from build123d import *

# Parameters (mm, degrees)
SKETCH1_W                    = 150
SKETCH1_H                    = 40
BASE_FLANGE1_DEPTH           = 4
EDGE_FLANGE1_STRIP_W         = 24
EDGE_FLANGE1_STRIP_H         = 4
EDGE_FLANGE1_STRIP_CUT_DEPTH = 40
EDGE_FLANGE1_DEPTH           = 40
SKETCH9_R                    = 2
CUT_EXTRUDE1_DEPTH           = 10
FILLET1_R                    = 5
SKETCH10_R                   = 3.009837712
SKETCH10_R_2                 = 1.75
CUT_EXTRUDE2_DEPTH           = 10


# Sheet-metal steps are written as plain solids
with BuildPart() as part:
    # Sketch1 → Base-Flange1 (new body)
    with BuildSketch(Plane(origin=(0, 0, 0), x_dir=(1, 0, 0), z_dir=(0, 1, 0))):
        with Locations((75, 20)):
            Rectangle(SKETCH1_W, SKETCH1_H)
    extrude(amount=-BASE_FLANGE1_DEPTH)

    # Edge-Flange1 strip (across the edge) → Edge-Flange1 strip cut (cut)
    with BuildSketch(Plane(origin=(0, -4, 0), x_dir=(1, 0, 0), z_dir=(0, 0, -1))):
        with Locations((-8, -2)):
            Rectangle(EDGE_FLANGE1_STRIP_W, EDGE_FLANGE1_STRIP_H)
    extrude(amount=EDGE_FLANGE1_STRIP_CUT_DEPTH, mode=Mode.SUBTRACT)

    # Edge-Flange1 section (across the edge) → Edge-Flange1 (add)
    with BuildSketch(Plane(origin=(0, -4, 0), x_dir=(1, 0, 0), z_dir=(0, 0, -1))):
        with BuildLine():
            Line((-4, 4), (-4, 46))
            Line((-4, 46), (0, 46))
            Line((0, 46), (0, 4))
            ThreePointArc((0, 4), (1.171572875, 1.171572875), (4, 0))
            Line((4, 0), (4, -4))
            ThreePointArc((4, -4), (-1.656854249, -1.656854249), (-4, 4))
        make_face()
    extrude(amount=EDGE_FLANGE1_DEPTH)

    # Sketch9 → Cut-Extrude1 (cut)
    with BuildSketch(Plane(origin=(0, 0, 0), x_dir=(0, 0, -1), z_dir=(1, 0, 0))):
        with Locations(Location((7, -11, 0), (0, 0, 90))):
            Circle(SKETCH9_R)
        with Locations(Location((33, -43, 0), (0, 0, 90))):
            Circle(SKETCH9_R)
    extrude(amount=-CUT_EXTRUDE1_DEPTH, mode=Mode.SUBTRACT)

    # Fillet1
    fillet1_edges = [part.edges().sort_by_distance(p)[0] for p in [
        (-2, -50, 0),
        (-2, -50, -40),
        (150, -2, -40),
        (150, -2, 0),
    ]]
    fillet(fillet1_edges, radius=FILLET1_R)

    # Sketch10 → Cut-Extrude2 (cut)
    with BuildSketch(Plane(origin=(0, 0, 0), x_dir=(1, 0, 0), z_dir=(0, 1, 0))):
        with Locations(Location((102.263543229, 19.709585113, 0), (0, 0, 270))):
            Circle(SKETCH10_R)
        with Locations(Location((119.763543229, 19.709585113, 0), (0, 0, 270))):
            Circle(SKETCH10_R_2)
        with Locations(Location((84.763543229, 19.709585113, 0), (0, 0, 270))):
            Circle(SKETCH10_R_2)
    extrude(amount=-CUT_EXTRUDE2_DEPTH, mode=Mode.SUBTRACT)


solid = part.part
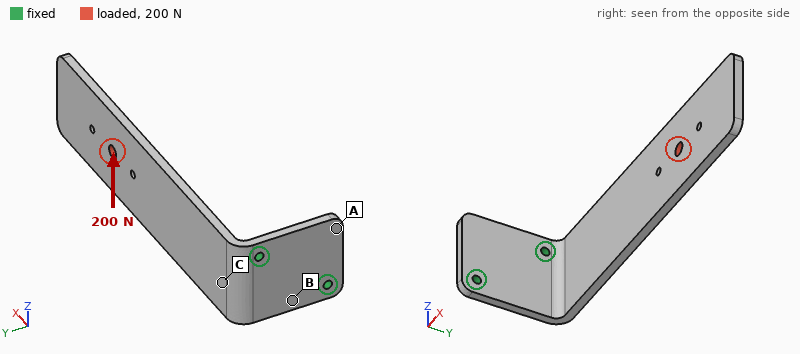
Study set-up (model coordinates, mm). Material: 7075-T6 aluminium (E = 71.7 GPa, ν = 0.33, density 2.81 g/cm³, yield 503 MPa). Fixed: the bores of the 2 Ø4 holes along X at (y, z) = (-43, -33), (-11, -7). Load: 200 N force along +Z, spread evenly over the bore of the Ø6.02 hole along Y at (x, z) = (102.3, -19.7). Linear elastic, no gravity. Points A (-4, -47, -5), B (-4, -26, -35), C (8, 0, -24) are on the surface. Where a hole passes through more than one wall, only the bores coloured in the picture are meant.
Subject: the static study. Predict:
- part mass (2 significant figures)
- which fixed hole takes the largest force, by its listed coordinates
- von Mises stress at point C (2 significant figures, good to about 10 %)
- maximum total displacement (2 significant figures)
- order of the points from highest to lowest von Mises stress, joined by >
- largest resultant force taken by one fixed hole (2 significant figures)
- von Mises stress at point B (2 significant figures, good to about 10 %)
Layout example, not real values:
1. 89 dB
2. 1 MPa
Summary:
1. 88 g
2. (-11, -7)
3. 36 MPa
4. 1.8 mm
5. B > C > A
6. 250 N
7. 59 MPa
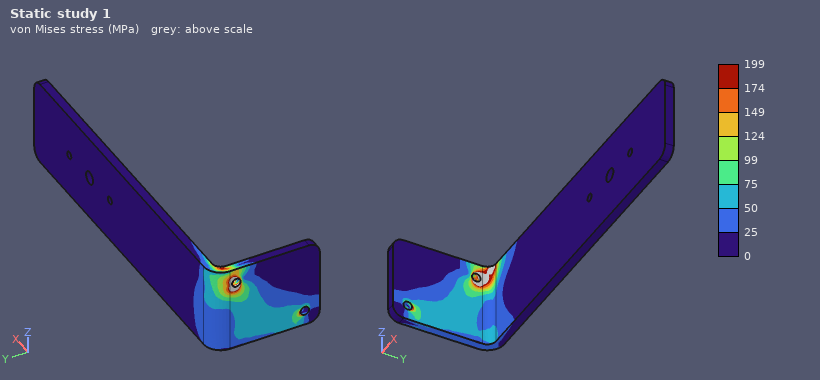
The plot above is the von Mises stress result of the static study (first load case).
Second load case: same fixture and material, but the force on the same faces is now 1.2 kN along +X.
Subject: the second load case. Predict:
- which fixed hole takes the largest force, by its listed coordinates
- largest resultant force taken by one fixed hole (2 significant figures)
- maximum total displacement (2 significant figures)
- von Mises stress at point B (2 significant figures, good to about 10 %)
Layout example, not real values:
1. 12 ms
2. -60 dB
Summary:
1. (-11, -7)
2. 1.2 kN
3. 1.6 mm
4. 49 MPa
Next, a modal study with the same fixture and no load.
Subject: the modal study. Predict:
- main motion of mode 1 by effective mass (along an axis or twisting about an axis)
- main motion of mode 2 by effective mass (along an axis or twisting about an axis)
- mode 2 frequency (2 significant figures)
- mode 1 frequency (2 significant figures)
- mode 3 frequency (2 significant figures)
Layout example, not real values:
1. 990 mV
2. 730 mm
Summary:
1. along Y
2. along Z
3. 310 Hz
4. 130 Hz
5. 820 Hz
